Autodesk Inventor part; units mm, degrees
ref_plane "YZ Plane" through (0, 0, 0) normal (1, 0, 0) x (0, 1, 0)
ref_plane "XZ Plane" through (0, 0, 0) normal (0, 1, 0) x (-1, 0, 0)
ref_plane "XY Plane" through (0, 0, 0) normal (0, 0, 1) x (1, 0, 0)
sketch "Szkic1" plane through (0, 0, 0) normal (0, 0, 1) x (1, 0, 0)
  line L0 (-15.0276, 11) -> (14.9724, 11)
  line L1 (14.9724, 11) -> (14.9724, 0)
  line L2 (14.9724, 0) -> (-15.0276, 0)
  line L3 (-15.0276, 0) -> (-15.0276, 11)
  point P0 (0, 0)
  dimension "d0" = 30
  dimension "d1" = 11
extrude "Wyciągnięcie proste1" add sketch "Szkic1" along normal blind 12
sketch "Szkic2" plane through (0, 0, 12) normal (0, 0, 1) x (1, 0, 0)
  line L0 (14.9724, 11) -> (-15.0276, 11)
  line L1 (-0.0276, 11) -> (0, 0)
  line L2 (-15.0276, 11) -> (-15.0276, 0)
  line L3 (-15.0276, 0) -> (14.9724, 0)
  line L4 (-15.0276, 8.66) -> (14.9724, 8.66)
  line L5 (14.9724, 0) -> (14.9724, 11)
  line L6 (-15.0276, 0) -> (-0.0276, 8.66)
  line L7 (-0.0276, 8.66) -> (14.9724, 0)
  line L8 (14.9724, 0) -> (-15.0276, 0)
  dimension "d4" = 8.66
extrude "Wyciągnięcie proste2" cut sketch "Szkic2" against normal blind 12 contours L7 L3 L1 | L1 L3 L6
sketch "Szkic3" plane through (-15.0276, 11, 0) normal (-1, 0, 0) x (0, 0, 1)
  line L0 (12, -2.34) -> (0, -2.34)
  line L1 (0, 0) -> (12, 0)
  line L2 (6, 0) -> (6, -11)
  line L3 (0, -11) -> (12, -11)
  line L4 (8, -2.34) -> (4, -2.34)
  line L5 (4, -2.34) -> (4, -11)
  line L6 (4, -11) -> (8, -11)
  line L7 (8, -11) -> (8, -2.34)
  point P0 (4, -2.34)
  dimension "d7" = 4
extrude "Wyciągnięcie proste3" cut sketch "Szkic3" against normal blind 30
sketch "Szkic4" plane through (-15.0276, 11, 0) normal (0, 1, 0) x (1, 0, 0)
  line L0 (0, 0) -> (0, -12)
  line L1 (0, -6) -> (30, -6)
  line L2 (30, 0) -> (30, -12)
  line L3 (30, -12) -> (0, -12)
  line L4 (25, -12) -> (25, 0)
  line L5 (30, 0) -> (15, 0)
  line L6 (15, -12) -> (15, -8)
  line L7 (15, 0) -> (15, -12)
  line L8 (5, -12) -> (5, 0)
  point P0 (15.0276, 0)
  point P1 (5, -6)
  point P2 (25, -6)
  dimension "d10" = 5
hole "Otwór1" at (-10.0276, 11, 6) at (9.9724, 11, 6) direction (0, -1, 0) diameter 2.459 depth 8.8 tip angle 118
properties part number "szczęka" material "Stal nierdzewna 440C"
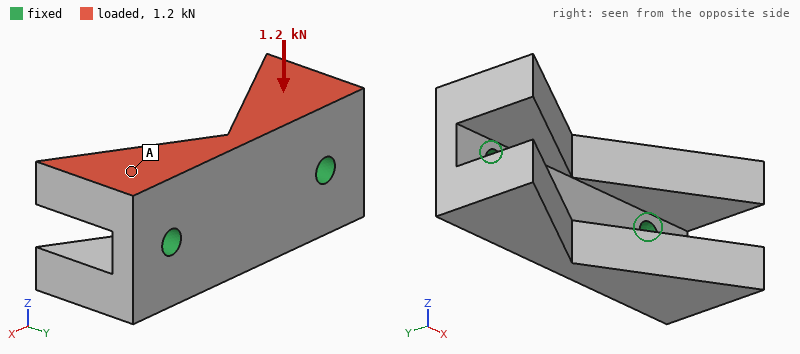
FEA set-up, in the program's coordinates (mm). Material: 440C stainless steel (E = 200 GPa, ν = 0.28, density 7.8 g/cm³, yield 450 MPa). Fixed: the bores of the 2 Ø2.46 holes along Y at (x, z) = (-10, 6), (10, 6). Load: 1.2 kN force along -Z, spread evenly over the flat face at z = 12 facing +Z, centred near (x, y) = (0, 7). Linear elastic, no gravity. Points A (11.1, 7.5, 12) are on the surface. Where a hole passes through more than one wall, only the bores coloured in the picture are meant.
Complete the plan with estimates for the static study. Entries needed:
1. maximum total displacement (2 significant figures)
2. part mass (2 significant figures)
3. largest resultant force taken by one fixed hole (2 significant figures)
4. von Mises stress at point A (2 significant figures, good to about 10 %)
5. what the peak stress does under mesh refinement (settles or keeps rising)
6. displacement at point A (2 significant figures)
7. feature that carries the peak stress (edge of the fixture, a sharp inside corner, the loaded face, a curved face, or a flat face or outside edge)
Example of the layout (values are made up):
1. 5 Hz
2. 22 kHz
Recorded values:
1. 23 µm
2. 15 g
3. 600 N
4. 32 MPa
5. keeps rising
6. 9.6 µm
7. edge of the fixture
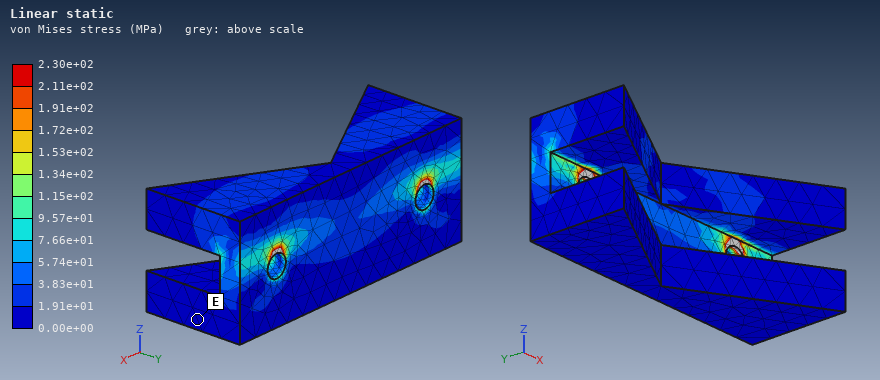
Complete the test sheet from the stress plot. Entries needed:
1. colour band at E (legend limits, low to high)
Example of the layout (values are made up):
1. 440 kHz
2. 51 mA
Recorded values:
1. 0.00e+00 to 1.91e+01 MPa
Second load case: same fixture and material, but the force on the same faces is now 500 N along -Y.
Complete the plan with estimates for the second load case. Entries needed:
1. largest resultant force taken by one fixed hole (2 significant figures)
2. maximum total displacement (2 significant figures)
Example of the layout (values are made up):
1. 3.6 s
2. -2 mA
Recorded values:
1. 250 N
2. 15 µm
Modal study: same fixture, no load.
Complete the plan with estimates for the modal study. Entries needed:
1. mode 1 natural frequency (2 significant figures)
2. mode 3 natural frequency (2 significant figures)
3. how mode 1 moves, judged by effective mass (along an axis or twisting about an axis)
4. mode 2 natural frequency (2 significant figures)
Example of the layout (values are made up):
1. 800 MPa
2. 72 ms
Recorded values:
1. 15 kHz
2. 20 kHz
3. along Z
4. 19 kHz
